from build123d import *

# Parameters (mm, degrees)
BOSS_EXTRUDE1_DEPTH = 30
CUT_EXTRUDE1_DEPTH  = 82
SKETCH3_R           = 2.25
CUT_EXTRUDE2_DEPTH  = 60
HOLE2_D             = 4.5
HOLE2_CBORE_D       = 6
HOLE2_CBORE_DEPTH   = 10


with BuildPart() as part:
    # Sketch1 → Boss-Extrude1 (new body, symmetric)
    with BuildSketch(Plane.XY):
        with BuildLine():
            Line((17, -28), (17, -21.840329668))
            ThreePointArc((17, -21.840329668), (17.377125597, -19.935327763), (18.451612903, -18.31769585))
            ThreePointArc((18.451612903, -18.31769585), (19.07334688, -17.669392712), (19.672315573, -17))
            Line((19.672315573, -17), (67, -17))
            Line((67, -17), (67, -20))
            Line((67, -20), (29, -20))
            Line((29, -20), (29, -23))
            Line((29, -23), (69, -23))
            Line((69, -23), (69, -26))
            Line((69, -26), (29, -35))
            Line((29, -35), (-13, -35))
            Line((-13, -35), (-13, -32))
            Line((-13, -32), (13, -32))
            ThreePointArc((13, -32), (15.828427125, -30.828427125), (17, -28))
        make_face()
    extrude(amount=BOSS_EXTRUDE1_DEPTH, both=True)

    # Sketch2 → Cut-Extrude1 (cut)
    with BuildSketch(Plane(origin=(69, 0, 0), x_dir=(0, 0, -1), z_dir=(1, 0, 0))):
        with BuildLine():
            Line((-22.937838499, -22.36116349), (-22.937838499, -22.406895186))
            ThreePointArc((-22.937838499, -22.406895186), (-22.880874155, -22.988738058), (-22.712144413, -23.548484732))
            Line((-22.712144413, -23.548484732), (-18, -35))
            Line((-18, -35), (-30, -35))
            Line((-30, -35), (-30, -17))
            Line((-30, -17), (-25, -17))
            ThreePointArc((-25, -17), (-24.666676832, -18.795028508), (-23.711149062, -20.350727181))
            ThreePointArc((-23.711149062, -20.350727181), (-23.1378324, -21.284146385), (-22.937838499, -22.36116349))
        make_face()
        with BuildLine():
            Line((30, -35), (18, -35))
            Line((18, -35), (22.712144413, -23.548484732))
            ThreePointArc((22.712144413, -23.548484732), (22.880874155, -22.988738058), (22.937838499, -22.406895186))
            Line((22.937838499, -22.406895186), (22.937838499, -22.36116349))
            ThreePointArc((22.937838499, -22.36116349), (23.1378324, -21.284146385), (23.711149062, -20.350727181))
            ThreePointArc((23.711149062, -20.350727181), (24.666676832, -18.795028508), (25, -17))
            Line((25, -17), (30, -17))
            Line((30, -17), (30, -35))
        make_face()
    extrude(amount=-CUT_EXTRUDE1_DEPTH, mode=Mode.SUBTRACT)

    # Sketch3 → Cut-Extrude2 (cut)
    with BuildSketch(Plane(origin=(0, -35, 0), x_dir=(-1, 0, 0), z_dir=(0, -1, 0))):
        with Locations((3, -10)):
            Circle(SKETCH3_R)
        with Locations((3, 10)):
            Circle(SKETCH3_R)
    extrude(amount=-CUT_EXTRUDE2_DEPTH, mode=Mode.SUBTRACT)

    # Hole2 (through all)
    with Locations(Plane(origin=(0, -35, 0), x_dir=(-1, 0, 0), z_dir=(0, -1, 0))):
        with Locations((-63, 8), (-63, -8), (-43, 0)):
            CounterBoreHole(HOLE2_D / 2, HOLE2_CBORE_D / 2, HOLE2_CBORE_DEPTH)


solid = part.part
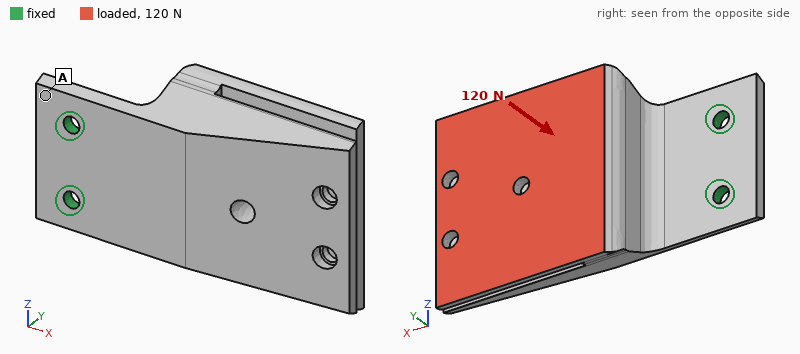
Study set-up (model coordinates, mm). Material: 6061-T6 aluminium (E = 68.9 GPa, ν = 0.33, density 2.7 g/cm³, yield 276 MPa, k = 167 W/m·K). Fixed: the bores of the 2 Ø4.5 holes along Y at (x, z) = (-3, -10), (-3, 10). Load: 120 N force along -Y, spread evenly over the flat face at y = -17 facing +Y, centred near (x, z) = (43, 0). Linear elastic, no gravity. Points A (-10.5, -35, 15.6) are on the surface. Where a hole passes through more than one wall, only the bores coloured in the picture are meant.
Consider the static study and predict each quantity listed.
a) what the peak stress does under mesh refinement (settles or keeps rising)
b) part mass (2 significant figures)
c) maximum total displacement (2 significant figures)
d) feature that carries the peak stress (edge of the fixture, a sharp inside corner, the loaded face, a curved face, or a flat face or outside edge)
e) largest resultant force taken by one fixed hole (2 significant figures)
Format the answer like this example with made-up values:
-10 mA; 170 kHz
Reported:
keeps rising; 82 g; 0.92 mm; edge of the fixture; 60 N
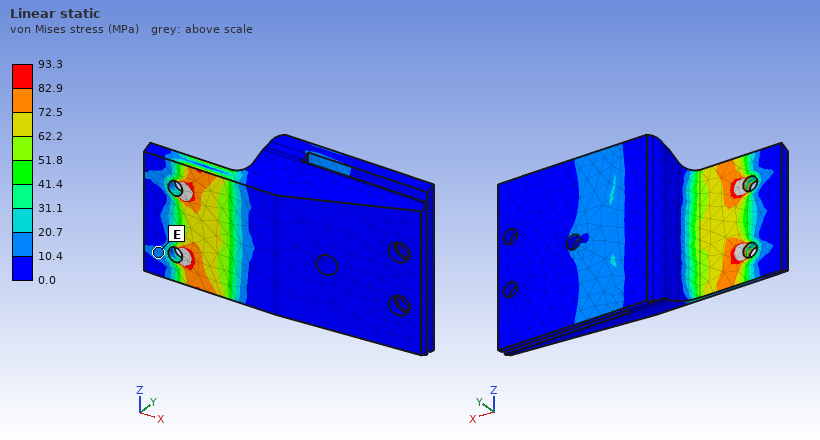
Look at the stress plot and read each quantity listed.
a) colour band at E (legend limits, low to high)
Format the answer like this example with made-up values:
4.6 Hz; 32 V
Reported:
10.4 to 20.7 MPa
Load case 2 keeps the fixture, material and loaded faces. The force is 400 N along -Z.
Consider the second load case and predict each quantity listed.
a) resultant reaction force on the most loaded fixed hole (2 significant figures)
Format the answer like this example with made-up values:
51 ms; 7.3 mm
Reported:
870 N
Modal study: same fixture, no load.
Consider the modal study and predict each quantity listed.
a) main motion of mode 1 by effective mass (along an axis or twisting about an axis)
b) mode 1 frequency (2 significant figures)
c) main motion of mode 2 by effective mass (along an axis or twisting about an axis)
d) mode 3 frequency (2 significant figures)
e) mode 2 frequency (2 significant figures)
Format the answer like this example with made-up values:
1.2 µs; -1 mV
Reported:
along Y; 300 Hz; along Z; 1900 Hz; 1300 Hz
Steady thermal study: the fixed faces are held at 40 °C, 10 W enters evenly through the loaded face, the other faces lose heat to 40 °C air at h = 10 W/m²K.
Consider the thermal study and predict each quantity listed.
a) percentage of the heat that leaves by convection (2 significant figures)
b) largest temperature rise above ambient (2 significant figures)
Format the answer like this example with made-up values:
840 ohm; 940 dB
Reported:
11 %; 18 K
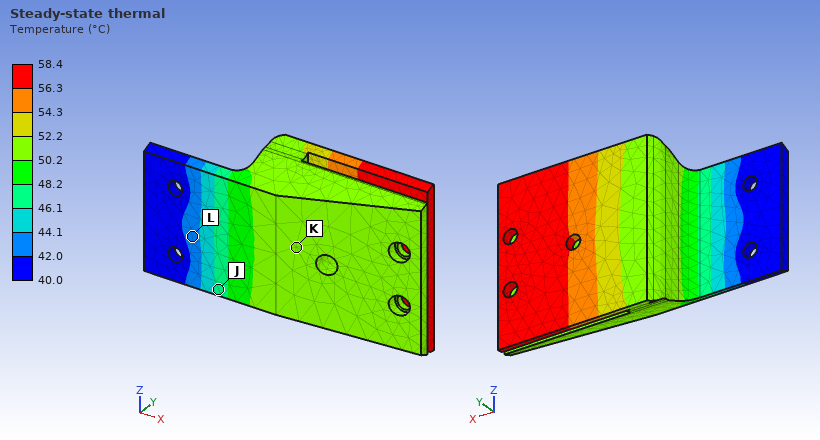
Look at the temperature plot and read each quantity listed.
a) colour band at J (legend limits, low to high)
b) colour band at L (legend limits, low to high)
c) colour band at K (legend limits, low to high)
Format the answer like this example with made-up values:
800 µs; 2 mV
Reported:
46.1 to 48.2 °C; 42.0 to 44.1 °C; 50.2 to 52.2 °C
